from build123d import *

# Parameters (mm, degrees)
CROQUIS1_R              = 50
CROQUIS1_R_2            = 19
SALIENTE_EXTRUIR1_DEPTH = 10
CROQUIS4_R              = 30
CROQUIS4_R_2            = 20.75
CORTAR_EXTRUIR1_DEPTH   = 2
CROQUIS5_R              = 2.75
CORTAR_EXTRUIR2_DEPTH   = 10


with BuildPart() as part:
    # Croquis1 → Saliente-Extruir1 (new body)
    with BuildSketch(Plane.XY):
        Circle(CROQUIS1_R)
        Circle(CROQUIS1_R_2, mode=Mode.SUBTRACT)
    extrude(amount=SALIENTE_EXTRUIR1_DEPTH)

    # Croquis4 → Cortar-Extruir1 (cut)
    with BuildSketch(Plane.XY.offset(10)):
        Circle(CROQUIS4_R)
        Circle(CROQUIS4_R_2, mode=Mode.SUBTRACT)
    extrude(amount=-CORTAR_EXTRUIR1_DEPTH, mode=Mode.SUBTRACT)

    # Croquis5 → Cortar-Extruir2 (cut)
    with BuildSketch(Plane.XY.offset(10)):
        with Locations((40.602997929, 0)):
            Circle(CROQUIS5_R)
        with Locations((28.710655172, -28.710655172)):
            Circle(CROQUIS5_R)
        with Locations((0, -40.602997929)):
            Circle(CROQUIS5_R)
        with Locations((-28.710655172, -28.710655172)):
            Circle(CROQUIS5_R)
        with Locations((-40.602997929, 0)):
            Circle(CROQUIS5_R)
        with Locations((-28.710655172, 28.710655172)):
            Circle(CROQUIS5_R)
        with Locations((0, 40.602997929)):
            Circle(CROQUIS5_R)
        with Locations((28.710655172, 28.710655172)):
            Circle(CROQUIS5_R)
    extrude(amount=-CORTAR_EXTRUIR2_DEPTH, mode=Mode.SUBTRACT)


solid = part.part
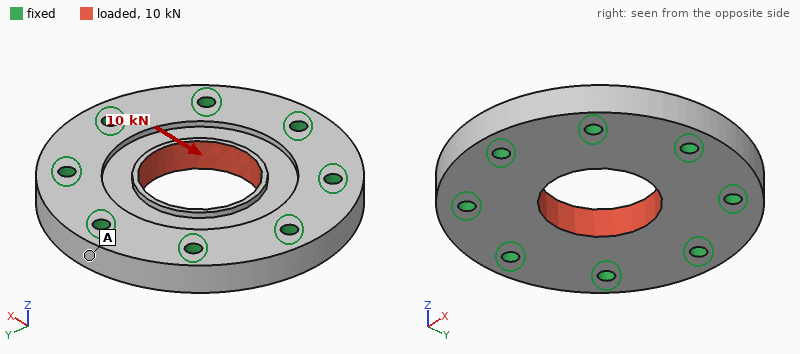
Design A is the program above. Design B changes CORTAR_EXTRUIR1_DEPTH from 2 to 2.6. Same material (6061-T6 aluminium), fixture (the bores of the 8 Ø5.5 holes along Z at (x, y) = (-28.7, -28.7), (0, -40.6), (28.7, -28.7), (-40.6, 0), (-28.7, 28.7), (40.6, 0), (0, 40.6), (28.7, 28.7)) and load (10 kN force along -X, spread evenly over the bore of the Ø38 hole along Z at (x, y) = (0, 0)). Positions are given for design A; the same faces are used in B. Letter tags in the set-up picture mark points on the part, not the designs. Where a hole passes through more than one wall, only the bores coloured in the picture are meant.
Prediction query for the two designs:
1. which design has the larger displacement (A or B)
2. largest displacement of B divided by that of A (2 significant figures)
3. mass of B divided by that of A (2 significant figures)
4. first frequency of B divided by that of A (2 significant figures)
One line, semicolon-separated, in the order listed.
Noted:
B; 1.3; 0.99; 1.0
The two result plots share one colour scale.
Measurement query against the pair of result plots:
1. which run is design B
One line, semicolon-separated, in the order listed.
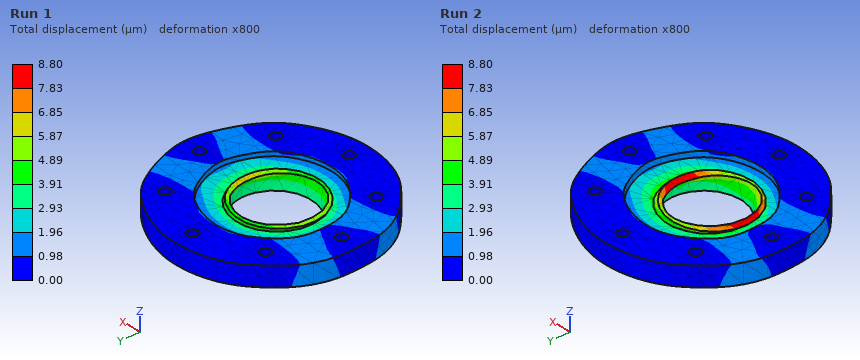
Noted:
Run 2
